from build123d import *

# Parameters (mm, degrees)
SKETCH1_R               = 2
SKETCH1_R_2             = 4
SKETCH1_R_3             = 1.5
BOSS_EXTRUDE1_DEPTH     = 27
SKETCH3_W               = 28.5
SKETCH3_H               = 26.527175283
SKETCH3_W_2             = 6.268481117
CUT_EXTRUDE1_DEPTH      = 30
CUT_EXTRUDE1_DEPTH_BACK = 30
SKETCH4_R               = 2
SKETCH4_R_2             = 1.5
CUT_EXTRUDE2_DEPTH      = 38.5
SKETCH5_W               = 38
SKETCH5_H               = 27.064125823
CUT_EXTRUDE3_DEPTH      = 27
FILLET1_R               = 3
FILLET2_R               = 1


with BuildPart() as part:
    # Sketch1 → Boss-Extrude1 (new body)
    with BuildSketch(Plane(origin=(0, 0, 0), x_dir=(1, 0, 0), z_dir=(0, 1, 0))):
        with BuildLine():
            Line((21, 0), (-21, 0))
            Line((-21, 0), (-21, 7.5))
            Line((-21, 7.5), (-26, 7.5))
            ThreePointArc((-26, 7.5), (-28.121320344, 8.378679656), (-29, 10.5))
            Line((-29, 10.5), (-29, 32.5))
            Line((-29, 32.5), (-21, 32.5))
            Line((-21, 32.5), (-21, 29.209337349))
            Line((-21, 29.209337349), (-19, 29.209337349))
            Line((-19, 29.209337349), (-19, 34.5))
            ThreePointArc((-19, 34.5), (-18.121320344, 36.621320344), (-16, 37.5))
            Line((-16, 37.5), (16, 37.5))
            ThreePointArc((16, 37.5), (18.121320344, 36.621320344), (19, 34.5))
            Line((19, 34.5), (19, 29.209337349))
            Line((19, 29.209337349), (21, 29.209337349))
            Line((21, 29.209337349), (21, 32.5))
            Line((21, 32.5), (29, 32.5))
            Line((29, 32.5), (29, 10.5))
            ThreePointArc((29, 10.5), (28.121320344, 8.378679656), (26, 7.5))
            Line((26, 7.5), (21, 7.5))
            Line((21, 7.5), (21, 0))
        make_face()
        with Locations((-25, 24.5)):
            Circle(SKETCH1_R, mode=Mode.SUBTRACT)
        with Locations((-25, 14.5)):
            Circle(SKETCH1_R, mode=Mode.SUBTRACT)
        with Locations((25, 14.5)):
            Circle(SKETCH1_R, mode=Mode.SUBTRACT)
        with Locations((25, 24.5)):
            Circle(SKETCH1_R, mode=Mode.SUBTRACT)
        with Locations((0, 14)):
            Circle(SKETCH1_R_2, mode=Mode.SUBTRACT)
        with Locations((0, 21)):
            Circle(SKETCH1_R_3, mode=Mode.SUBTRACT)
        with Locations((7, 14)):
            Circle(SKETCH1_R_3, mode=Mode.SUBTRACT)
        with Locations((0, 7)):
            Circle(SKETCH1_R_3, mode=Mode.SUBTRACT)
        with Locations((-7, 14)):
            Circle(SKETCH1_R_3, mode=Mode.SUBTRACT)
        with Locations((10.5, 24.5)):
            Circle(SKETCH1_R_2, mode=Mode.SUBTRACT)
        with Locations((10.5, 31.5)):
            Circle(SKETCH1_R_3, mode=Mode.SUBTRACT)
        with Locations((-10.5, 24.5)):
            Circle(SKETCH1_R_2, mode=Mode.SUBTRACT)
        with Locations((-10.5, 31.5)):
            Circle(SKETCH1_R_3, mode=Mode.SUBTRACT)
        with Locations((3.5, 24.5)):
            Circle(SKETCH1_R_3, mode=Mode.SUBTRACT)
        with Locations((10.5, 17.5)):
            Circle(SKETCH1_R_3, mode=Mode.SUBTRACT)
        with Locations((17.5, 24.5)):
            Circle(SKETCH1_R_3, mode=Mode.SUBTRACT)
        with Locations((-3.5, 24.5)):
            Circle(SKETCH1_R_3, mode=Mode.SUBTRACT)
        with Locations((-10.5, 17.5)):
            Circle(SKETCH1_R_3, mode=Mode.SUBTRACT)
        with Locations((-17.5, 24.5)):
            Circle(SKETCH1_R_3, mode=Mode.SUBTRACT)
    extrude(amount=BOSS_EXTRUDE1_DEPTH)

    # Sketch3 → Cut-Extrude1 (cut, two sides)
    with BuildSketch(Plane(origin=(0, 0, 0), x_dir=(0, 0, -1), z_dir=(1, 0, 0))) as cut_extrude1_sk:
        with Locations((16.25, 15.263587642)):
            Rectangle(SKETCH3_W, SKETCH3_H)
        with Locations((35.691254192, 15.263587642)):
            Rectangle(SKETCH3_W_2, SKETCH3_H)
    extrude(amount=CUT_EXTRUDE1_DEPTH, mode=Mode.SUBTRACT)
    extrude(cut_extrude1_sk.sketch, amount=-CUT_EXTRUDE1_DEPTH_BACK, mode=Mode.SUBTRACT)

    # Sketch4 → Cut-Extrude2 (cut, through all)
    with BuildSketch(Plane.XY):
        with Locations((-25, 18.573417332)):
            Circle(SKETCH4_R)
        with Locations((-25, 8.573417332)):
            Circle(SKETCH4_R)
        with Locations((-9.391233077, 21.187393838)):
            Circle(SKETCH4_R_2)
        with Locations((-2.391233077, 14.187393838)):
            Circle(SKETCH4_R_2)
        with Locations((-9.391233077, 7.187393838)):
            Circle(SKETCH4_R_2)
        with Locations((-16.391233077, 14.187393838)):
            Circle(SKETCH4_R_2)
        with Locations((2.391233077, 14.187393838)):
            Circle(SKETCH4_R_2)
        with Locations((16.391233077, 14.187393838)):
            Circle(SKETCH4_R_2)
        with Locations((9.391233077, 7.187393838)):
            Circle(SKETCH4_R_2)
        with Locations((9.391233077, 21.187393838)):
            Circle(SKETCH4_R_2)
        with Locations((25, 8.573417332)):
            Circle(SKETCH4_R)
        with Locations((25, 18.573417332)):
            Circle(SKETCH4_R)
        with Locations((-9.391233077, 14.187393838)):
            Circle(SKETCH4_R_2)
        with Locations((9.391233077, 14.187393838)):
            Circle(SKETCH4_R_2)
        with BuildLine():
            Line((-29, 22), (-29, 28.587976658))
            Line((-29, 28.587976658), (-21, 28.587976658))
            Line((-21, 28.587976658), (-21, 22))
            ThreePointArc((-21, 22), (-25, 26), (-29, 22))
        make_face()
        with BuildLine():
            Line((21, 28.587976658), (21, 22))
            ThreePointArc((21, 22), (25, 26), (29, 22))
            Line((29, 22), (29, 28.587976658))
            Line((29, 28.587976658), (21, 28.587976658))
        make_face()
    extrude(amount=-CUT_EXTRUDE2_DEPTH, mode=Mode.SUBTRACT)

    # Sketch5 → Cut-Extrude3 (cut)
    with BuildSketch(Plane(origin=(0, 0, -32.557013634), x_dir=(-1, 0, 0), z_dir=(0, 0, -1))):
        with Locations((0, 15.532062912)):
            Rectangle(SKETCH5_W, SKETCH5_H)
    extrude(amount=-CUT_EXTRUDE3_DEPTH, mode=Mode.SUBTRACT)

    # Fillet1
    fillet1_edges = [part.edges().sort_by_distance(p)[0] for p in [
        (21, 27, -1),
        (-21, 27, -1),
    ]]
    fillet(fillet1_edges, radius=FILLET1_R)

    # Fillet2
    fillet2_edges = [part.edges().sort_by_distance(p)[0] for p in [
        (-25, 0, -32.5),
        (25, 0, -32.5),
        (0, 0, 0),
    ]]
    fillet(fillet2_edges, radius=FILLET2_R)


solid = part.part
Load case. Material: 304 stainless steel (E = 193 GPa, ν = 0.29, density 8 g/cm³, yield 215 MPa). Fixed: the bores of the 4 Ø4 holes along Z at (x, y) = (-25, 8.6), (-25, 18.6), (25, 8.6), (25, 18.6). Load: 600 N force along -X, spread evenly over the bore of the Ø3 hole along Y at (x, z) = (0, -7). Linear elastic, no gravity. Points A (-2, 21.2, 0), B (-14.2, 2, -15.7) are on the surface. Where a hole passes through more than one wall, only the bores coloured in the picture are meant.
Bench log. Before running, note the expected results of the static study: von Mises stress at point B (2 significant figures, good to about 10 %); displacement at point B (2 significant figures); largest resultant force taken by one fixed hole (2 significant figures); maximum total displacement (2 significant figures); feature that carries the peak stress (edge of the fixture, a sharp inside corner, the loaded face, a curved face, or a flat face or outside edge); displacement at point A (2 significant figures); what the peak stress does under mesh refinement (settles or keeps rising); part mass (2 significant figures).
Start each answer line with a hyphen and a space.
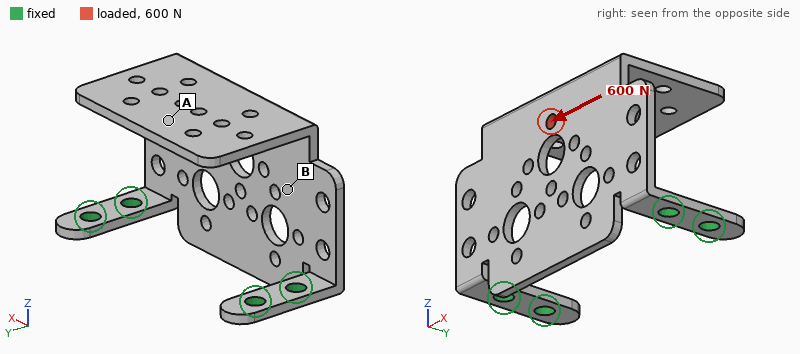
- 30 MPa
- 30 µm
- 440 N
- 82 µm
- edge of the fixture
- 66 µm
- keeps rising
- 47 g
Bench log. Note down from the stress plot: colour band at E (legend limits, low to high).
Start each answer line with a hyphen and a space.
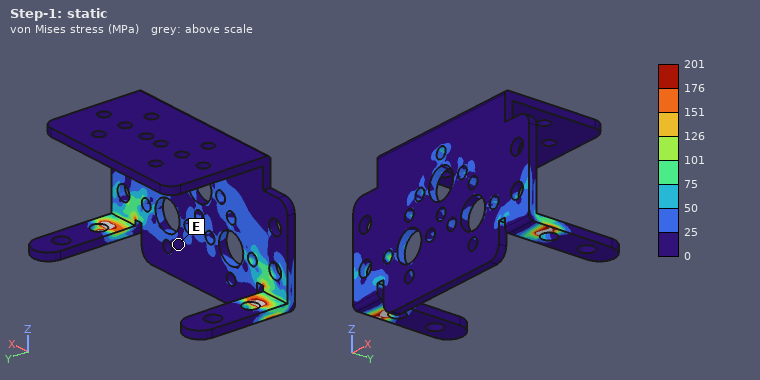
- 0 to 25 MPa
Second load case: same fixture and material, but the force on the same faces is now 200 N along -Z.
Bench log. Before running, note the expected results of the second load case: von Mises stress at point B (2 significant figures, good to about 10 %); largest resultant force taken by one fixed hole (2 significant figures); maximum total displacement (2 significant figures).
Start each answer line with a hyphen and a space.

- 5.2 MPa
- 100 N
- 68 µm
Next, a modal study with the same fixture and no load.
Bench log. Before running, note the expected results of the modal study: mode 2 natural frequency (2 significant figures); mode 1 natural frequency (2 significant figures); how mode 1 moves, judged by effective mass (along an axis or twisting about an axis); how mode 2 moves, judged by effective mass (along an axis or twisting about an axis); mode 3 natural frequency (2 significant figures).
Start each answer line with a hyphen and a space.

- 1100 Hz
- 380 Hz
- along Y
- along X
- 1500 Hz
